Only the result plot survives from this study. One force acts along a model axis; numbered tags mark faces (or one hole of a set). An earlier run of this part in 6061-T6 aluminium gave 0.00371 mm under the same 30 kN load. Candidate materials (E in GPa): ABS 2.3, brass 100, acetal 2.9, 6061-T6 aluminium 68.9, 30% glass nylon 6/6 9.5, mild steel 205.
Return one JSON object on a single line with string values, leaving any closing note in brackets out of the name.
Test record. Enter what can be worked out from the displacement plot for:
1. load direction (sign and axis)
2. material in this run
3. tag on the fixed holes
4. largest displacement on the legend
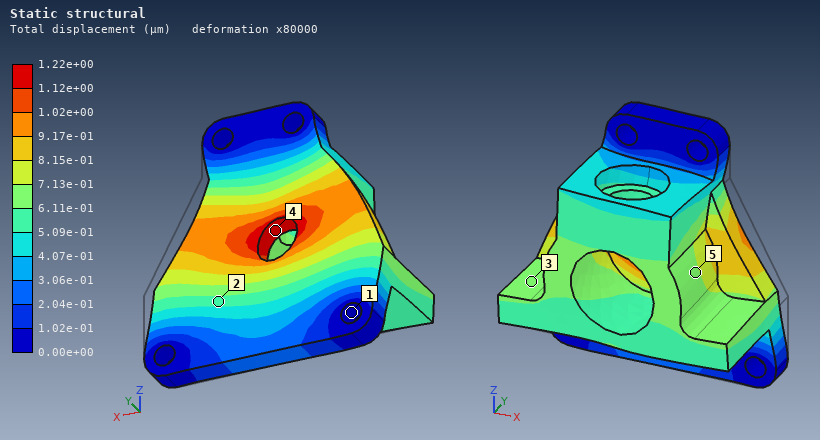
{"load direction": "-X", "material in this run": "mild steel", "tag on the fixed holes": "1", "largest displacement on the legend": "1.22e+00 µm"}
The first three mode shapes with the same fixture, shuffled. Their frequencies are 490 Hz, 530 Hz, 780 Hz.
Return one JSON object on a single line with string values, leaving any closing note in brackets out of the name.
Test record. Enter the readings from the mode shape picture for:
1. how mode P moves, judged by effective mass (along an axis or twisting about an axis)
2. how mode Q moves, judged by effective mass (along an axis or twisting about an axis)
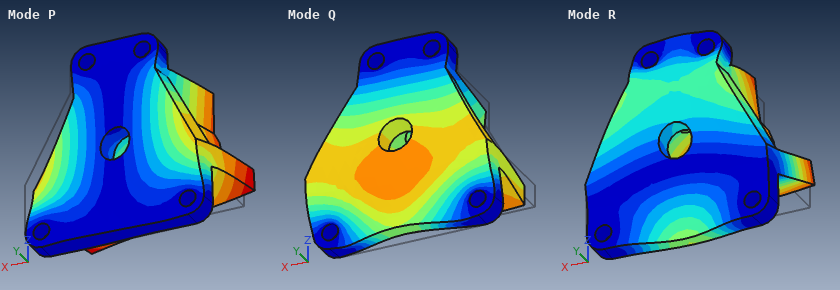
{"how mode P moves, judged by effective mass": "along X", "how mode Q moves, judged by effective mass": "along Y"}
